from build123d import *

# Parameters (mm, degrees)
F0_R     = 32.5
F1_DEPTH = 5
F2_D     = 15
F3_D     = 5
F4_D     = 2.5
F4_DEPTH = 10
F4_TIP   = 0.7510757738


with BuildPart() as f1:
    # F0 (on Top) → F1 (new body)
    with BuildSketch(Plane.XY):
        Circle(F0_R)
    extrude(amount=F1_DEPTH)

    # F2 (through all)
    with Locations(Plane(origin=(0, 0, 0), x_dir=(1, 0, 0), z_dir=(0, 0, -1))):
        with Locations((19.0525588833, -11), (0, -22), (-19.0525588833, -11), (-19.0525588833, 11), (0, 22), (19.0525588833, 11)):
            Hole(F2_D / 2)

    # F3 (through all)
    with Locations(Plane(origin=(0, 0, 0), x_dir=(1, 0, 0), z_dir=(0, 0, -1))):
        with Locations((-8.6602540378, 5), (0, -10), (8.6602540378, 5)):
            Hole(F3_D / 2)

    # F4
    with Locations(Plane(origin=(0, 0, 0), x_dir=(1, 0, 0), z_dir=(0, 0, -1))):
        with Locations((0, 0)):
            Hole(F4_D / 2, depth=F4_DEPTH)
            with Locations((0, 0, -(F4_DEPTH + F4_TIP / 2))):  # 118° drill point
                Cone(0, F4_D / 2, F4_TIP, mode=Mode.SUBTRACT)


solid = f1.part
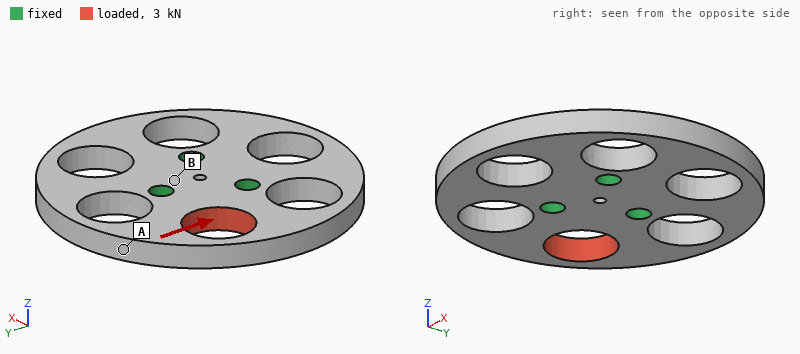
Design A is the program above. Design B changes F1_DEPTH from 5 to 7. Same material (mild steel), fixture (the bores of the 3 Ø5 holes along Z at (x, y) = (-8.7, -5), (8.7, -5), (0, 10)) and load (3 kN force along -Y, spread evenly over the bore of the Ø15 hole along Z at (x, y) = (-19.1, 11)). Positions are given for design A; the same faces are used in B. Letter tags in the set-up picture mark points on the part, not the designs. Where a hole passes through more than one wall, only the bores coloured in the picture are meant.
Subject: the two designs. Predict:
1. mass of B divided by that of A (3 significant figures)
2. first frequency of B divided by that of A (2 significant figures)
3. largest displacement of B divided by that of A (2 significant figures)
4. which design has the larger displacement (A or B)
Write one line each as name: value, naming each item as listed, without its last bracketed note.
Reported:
mass of B divided by that of A: 1.40
first frequency of B divided by that of A: 1.3
largest displacement of B divided by that of A: 0.70
which design has the larger displacement: A
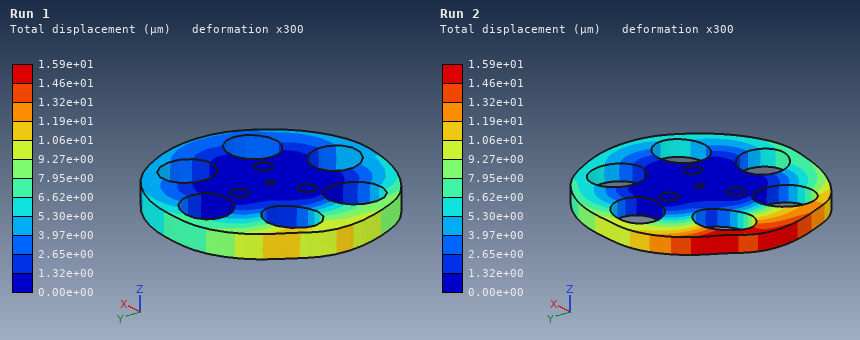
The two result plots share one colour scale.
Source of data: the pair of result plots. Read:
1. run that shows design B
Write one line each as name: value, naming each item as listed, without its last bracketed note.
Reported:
run that shows design B: Run 1
